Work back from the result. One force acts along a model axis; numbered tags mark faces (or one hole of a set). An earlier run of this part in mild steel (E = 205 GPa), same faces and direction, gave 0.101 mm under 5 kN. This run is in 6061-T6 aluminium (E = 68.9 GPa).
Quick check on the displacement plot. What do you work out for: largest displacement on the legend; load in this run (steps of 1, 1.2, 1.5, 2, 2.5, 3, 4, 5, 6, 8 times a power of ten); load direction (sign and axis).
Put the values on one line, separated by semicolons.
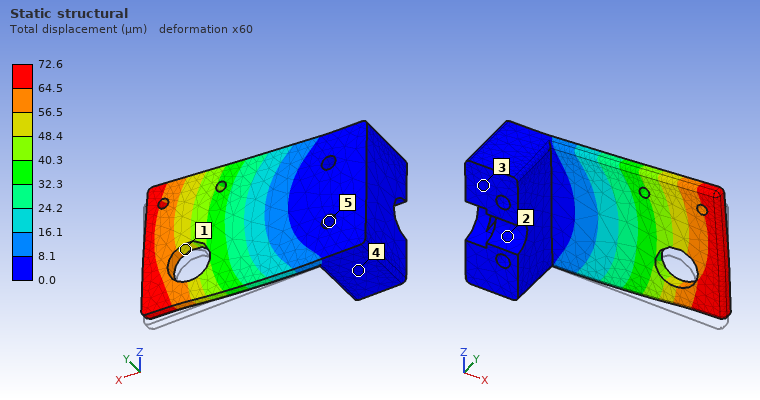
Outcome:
72.6 µm; 1.2 kN; +Z
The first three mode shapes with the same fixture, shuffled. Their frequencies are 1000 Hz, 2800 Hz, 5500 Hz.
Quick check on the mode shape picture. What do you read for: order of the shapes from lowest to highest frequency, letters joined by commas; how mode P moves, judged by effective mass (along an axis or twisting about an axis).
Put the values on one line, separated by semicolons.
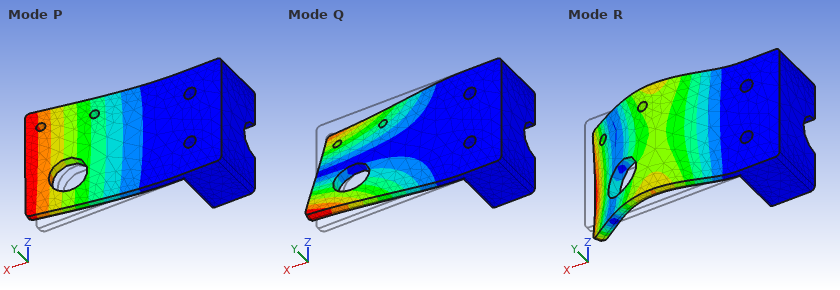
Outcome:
P, Q, R; along Y
